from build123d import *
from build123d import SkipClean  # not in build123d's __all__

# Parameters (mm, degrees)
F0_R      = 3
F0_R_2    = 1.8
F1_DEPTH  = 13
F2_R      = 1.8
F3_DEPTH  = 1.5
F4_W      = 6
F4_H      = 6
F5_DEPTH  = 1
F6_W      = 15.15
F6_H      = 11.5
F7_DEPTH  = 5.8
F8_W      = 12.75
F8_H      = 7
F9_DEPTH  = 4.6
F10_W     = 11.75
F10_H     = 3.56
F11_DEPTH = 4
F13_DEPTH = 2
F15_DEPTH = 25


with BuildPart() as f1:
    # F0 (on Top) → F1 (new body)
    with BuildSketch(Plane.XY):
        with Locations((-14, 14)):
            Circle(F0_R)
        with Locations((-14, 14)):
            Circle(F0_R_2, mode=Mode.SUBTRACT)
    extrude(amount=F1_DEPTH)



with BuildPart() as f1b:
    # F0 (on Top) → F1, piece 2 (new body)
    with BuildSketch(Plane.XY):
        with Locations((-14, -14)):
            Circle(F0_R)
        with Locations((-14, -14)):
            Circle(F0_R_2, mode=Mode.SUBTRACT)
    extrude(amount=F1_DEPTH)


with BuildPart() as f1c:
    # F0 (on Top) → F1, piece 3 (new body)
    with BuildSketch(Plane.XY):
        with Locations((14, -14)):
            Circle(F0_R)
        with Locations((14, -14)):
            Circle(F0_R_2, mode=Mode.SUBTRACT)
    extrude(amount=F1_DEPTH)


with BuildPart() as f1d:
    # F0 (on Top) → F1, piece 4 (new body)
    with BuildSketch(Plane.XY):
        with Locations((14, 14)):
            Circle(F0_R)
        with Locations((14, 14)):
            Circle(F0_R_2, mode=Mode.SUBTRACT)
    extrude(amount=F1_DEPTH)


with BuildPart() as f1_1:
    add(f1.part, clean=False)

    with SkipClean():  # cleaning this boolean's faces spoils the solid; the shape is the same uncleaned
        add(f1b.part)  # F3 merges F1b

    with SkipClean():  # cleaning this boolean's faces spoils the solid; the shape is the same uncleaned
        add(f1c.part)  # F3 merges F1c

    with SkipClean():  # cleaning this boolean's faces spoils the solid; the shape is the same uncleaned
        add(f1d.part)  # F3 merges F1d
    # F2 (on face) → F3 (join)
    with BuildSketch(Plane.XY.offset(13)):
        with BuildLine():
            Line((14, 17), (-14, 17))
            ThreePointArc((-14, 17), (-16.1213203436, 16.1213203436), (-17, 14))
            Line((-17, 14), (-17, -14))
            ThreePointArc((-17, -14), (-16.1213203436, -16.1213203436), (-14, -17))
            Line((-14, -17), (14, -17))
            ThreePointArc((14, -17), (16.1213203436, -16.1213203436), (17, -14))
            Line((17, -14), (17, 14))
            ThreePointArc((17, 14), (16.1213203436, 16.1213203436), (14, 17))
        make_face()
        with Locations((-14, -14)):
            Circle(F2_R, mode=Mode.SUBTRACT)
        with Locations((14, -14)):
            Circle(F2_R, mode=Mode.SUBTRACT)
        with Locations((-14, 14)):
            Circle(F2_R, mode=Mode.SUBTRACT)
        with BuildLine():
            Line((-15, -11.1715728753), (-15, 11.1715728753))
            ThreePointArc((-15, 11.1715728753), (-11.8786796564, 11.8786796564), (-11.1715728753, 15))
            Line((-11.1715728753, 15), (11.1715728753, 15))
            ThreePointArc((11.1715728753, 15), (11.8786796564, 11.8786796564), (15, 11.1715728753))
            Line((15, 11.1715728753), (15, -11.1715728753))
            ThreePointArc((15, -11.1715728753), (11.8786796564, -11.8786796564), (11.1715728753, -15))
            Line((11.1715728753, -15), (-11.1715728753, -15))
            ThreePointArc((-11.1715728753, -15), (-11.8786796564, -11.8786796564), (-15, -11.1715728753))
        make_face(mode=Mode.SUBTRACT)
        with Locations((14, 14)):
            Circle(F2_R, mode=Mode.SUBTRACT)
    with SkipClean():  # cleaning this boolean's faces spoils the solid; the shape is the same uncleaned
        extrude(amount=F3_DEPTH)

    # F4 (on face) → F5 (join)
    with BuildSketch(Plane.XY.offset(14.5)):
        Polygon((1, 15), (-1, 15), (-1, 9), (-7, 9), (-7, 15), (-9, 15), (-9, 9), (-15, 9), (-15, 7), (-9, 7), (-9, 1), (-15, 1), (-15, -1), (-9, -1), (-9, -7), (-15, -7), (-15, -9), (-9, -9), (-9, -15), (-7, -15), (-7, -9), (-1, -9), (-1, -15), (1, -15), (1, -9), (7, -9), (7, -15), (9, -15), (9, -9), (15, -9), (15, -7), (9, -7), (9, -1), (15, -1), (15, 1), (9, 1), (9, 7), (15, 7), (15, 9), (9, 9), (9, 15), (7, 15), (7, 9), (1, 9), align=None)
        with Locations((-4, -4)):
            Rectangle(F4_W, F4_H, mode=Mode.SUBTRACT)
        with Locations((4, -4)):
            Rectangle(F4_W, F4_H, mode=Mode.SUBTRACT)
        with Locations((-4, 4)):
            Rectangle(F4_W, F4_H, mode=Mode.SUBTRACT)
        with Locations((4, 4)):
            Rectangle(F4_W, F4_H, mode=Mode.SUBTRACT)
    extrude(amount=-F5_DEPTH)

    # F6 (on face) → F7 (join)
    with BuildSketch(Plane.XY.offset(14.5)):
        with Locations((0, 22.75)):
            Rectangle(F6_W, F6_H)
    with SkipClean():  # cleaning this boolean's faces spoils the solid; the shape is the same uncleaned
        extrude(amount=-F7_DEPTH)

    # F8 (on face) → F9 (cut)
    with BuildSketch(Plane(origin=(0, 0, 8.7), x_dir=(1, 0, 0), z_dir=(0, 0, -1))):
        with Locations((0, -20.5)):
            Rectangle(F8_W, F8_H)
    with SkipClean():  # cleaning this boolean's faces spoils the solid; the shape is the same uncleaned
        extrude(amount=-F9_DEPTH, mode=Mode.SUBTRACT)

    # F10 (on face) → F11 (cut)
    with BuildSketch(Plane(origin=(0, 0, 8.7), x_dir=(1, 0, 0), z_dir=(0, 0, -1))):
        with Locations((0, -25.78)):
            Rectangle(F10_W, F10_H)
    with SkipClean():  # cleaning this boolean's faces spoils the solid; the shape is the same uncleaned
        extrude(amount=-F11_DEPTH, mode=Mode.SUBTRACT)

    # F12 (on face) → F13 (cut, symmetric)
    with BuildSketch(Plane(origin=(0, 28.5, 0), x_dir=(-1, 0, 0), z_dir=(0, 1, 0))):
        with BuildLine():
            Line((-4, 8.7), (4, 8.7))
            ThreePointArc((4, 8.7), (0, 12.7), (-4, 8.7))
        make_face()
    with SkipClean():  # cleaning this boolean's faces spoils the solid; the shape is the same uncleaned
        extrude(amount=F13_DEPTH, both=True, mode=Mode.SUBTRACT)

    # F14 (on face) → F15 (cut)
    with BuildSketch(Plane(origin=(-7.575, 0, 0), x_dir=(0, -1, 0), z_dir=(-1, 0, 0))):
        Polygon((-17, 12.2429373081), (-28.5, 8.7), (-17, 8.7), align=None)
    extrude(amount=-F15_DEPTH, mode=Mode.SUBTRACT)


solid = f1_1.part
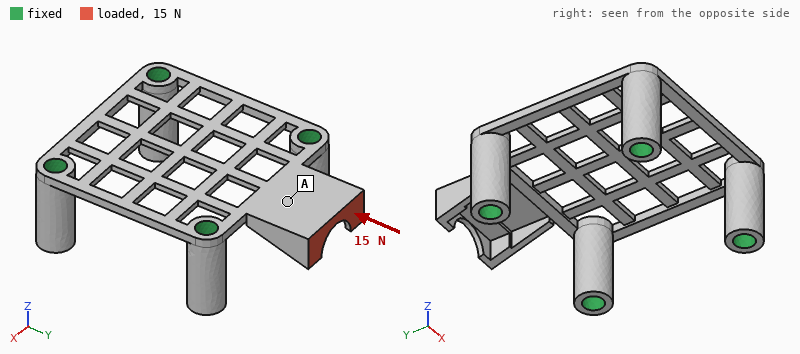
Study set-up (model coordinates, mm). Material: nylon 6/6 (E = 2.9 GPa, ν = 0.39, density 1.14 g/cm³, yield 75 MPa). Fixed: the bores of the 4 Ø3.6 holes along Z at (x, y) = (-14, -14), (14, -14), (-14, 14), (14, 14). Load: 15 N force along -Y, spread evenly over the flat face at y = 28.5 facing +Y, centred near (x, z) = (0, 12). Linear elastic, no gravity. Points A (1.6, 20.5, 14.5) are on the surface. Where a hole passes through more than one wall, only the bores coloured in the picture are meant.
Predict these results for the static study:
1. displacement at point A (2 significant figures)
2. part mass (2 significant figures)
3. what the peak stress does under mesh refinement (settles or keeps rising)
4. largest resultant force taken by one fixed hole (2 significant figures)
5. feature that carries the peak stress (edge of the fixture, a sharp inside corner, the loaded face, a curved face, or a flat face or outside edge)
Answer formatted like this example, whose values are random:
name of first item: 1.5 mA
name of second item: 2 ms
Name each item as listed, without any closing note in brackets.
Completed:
displacement at point A: 0.19 mm
part mass: 2.3 g
what the peak stress does under mesh refinement: keeps rising
largest resultant force taken by one fixed hole: 6.2 N
feature that carries the peak stress: a sharp inside corner
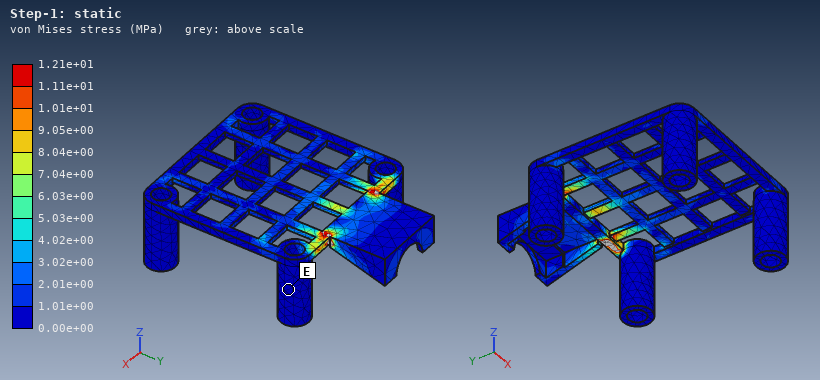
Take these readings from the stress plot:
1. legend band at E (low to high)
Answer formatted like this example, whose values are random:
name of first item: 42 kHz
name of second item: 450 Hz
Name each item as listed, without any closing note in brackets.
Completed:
legend band at E: 0.00e+00 to 1.01e+00 MPa
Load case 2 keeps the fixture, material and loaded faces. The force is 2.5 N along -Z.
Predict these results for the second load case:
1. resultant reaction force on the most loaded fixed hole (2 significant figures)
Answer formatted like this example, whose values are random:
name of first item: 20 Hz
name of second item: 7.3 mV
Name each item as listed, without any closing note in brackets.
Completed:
resultant reaction force on the most loaded fixed hole: 1.7 N
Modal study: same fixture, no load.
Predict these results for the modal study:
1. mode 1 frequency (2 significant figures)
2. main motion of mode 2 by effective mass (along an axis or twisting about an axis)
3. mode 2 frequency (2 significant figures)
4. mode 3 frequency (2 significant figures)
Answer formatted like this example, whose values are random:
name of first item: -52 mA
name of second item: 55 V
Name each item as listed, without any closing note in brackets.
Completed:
mode 1 frequency: 700 Hz
main motion of mode 2 by effective mass: along Z
mode 2 frequency: 1500 Hz
mode 3 frequency: 2600 Hz
